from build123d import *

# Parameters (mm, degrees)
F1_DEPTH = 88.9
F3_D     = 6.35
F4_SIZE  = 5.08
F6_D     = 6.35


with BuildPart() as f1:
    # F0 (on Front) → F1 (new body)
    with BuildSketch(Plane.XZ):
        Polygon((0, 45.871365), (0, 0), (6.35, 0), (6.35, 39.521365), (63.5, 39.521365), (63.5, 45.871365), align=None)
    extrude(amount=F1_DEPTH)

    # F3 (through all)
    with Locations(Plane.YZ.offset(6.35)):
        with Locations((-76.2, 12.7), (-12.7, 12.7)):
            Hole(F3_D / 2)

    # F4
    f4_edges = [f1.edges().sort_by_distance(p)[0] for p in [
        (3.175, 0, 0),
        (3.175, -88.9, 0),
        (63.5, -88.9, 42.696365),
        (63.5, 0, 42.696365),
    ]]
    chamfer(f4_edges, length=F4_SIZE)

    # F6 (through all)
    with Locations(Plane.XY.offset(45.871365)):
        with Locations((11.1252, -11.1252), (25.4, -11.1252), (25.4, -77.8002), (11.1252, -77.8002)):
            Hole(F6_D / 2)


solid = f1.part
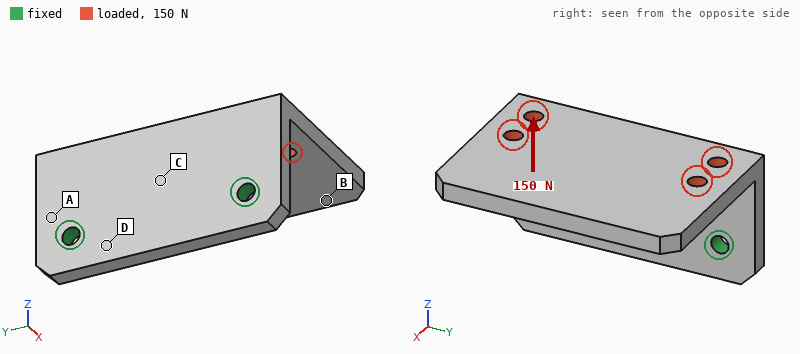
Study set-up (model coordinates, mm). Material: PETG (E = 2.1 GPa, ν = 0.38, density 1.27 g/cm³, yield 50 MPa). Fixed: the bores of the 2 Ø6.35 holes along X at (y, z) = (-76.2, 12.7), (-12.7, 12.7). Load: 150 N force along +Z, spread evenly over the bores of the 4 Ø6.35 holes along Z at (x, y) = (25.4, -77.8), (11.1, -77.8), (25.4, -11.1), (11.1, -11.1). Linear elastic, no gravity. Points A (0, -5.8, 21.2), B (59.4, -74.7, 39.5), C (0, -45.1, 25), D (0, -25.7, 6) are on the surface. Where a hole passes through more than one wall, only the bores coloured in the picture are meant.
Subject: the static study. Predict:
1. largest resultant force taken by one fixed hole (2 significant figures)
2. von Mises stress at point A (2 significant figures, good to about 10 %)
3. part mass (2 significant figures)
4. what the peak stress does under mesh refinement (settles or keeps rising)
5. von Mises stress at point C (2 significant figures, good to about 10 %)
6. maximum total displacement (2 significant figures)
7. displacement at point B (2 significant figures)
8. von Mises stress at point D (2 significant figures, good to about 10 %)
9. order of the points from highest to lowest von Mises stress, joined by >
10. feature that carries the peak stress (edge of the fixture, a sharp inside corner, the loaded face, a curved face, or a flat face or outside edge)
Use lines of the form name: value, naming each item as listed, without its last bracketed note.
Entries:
largest resultant force taken by one fixed hole: 76 N
von Mises stress at point A: 4.0 MPa
part mass: 72 g
what the peak stress does under mesh refinement: keeps rising
von Mises stress at point C: 2.4 MPa
maximum total displacement: 1.3 mm
displacement at point B: 1.2 mm
von Mises stress at point D: 1.3 MPa
order of the points from highest to lowest von Mises stress, joined by >: A > C > D > B
feature that carries the peak stress: edge of the fixture
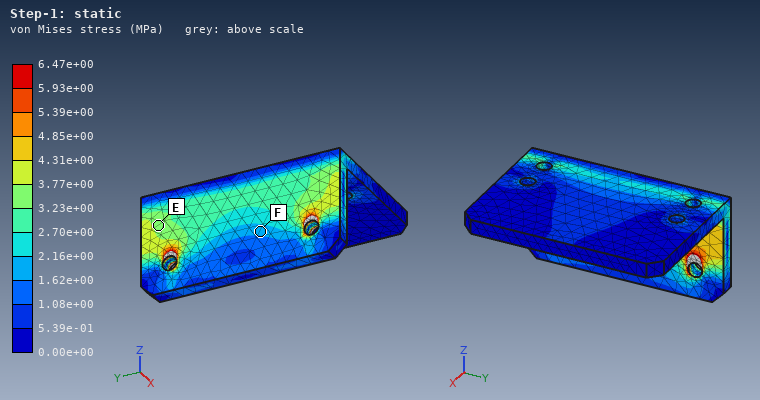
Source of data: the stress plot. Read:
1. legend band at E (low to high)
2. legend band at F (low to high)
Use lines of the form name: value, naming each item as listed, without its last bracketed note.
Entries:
legend band at E: 3.23e+00 to 3.77e+00 MPa
legend band at F: 1.62e+00 to 2.16e+00 MPa
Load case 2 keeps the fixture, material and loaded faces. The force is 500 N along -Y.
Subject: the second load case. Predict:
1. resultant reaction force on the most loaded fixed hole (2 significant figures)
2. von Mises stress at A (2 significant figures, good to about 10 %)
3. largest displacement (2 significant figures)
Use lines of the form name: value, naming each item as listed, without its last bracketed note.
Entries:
resultant reaction force on the most loaded fixed hole: 350 N
von Mises stress at A: 6.7 MPa
largest displacement: 0.87 mm
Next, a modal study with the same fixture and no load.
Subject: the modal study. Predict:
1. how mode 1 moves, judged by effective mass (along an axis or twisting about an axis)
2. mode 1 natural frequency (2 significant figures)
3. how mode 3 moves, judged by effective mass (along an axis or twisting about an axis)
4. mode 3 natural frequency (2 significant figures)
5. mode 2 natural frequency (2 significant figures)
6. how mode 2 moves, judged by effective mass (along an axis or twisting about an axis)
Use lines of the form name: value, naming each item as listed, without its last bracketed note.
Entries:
how mode 1 moves, judged by effective mass: along Z
mode 1 natural frequency: 200 Hz
how mode 3 moves, judged by effective mass: along X
mode 3 natural frequency: 630 Hz
mode 2 natural frequency: 420 Hz
how mode 2 moves, judged by effective mass: along Y
